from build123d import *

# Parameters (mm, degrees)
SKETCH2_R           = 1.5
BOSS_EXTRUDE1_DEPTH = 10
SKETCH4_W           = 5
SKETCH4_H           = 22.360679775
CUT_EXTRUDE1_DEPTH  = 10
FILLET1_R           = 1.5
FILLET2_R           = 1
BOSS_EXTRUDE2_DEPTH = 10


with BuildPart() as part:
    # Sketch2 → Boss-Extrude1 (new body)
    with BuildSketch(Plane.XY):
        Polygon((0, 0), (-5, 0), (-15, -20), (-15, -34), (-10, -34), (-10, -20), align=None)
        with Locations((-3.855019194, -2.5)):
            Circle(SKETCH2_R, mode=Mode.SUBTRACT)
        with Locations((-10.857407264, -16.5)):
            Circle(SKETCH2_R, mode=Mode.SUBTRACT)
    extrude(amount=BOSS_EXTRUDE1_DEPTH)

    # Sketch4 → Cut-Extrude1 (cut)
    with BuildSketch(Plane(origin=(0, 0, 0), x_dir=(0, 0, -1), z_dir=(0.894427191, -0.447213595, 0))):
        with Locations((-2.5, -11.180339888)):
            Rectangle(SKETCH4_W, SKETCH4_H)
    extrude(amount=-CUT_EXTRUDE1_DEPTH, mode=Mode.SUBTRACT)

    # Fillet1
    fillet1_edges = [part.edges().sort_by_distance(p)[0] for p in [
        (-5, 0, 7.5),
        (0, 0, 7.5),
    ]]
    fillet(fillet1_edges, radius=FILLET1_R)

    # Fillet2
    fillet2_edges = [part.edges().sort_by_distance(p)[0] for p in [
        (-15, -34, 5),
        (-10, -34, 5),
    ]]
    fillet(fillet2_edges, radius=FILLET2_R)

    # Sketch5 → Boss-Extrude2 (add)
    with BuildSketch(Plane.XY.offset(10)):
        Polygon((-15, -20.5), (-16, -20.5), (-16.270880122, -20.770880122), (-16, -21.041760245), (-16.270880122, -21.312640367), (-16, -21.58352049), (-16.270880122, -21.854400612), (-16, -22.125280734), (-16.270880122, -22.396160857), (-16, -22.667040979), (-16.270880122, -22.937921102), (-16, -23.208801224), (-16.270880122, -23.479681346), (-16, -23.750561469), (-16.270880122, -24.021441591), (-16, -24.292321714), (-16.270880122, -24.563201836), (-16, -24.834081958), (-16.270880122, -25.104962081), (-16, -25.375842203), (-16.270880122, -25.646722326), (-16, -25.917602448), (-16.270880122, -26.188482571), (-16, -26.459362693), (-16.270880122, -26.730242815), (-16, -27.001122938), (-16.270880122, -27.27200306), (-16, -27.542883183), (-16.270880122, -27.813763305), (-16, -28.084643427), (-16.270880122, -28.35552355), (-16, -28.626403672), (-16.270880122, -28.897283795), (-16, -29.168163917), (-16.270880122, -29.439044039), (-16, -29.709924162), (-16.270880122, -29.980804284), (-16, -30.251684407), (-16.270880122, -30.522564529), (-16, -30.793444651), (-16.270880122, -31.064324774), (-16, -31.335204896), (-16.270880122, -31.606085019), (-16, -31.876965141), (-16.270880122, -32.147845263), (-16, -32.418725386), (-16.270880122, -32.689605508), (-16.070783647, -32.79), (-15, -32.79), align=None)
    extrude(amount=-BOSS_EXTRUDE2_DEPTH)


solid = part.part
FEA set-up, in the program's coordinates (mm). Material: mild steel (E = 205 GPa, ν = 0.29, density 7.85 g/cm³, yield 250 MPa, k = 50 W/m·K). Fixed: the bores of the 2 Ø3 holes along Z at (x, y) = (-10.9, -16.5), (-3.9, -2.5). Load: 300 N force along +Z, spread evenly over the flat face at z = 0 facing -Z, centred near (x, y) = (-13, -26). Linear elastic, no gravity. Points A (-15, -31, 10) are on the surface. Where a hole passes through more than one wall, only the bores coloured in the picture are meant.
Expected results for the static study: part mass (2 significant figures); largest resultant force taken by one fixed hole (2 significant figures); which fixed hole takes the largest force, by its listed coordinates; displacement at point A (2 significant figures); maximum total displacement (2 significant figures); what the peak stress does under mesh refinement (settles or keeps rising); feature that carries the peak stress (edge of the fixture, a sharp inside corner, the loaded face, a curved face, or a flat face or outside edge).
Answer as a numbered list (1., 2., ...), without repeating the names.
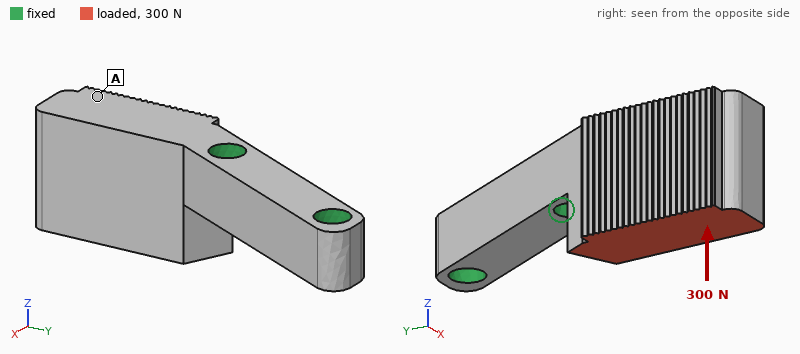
1. 10 g
2. 300 N
3. (-10.9, -16.5)
4. 13 µm
5. 17 µm
6. keeps rising
7. edge of the fixture
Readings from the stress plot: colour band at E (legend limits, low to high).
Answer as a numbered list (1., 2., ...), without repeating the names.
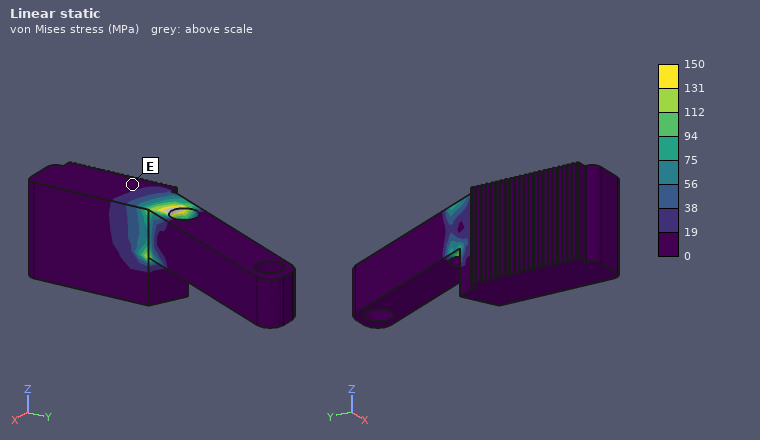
1. 0 to 19 MPa
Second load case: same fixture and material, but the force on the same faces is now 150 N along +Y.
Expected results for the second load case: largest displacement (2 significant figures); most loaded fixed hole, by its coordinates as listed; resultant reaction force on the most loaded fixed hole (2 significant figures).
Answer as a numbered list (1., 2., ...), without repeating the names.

1. 8.4 µm
2. (-10.9, -16.5)
3. 150 N
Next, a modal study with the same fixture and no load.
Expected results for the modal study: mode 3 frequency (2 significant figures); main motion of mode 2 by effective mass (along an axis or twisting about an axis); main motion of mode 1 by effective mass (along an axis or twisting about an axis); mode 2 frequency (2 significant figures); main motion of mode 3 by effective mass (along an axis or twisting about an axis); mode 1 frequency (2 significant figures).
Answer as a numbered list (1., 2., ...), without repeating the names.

1. 21 kHz
2. along Z
3. along X
4. 9700 Hz
5. twisting about Y
6. 8300 Hz
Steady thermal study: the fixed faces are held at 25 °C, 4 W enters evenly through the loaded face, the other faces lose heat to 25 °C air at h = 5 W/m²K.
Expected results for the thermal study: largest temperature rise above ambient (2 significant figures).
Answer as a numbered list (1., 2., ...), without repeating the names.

1. 24 K
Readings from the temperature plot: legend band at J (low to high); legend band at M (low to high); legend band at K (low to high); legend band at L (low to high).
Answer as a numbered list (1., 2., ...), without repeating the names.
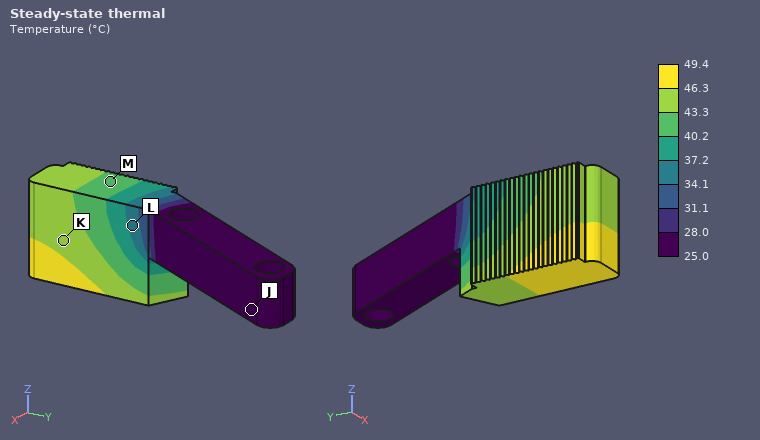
1. 25.0 to 28.0 °C
2. 40.2 to 43.3 °C
3. 43.3 to 46.3 °C
4. 34.1 to 37.2 °C
